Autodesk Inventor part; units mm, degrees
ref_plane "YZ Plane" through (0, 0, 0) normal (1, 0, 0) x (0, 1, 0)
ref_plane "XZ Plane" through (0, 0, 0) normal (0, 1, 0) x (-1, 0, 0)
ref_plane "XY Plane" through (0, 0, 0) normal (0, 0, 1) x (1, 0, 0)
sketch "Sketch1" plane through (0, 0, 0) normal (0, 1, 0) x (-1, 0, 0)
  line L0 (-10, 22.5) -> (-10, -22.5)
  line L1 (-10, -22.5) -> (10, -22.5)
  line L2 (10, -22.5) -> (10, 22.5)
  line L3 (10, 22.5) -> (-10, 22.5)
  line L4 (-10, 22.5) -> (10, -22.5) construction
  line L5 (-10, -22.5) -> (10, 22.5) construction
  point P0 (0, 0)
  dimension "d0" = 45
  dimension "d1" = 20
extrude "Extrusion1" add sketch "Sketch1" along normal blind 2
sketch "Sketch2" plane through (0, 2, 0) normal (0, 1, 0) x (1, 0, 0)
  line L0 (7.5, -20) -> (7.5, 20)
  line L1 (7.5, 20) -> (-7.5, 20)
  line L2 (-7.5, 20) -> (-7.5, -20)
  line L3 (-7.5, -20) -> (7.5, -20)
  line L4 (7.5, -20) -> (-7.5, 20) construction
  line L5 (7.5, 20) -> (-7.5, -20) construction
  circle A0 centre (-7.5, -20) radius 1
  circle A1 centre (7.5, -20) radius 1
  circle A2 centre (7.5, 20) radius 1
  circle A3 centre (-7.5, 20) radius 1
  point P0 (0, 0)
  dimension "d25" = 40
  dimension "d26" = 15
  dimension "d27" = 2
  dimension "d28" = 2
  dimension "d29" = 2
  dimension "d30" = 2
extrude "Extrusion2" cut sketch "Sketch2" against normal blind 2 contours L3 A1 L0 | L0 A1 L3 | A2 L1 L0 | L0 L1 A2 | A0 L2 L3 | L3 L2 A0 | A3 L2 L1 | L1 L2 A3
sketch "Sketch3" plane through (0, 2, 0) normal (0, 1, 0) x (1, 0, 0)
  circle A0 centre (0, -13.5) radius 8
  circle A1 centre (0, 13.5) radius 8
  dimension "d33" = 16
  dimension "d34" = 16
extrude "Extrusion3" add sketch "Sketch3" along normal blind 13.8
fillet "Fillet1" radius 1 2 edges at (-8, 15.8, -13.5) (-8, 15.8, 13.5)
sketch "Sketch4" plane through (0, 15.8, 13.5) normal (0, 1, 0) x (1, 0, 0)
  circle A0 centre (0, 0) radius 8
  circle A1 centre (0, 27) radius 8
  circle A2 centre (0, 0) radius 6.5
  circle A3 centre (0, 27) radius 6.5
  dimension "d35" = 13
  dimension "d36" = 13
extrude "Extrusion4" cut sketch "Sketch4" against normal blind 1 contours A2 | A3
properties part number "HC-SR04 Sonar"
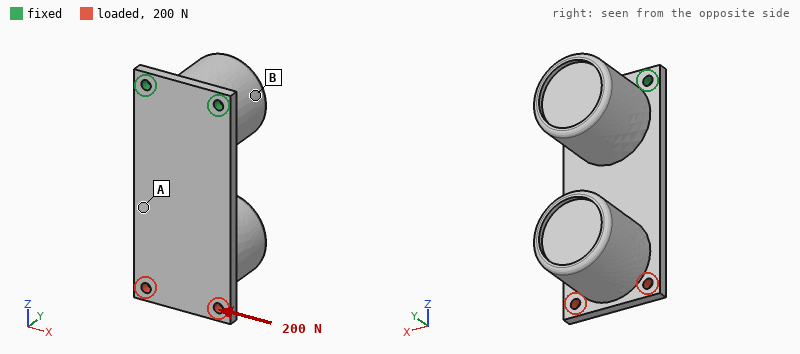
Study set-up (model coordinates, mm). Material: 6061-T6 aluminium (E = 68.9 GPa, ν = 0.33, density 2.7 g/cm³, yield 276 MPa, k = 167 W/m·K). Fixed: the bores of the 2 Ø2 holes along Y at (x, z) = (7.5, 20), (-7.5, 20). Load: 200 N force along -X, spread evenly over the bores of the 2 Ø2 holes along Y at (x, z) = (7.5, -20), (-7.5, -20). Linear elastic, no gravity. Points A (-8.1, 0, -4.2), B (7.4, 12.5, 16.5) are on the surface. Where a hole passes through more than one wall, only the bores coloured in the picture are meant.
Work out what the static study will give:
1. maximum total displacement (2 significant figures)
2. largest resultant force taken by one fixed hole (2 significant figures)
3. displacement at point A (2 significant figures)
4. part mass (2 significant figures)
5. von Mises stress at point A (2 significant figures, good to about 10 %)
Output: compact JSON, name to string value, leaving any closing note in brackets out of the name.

{"maximum total displacement": "56 µm", "largest resultant force taken by one fixed hole": "530 N", "displacement at point A": "25 µm", "part mass": "19 g", "von Mises stress at point A": "18 MPa"}
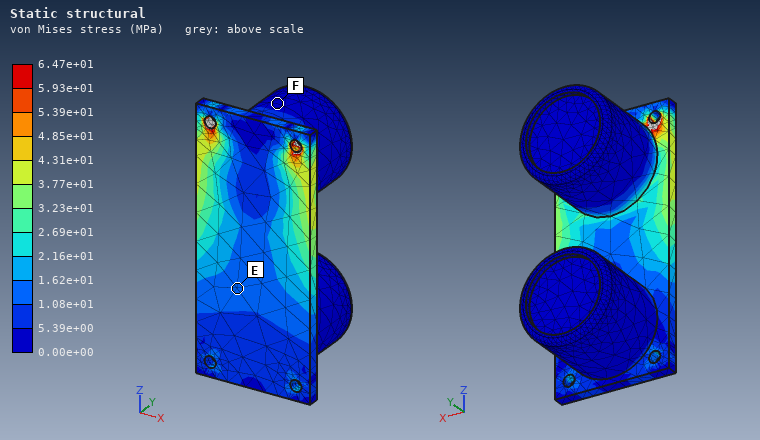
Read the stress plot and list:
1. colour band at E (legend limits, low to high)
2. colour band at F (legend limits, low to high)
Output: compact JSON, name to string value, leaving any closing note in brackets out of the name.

{"colour band at E": "1.08e+01 to 1.62e+01 MPa", "colour band at F": "0.00e+00 to 5.39e+00 MPa"}
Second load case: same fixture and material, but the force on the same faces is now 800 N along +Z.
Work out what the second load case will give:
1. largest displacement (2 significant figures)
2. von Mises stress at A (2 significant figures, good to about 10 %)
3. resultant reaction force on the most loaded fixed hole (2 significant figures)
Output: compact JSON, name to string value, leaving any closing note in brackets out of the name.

{"largest displacement": "29 µm", "von Mises stress at A": "20 MPa", "resultant reaction force on the most loaded fixed hole": "410 N"}
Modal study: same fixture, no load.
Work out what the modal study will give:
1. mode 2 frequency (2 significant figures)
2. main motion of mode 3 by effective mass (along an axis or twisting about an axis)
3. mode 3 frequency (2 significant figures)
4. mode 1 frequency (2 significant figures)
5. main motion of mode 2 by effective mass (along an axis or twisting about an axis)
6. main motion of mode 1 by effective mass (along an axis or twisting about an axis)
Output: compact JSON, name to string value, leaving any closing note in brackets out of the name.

{"mode 2 frequency": "2100 Hz", "main motion of mode 3 by effective mass": "along Y", "mode 3 frequency": "2800 Hz", "mode 1 frequency": "620 Hz", "main motion of mode 2 by effective mass": "along X", "main motion of mode 1 by effective mass": "along Y"}
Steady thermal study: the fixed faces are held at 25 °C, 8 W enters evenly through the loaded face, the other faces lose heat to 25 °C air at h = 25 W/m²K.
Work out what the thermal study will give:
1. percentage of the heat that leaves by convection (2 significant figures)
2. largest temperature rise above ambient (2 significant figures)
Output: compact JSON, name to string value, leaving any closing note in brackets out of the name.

{"percentage of the heat that leaves by convection": "17 %", "largest temperature rise above ambient": "35 K"}
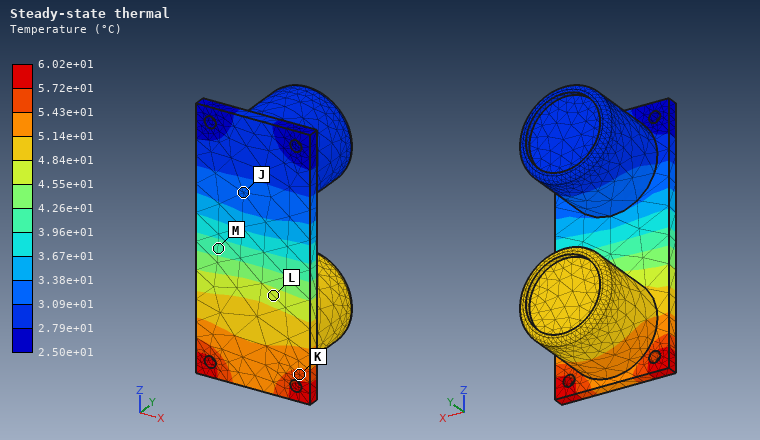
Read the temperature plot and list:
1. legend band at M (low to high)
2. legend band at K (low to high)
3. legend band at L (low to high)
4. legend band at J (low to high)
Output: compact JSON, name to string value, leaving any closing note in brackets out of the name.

{"legend band at M": "3.96e+01 to 4.26e+01 °C", "legend band at K": "5.43e+01 to 5.72e+01 °C", "legend band at L": "4.55e+01 to 4.84e+01 °C", "legend band at J": "3.09e+01 to 3.38e+01 °C"}
